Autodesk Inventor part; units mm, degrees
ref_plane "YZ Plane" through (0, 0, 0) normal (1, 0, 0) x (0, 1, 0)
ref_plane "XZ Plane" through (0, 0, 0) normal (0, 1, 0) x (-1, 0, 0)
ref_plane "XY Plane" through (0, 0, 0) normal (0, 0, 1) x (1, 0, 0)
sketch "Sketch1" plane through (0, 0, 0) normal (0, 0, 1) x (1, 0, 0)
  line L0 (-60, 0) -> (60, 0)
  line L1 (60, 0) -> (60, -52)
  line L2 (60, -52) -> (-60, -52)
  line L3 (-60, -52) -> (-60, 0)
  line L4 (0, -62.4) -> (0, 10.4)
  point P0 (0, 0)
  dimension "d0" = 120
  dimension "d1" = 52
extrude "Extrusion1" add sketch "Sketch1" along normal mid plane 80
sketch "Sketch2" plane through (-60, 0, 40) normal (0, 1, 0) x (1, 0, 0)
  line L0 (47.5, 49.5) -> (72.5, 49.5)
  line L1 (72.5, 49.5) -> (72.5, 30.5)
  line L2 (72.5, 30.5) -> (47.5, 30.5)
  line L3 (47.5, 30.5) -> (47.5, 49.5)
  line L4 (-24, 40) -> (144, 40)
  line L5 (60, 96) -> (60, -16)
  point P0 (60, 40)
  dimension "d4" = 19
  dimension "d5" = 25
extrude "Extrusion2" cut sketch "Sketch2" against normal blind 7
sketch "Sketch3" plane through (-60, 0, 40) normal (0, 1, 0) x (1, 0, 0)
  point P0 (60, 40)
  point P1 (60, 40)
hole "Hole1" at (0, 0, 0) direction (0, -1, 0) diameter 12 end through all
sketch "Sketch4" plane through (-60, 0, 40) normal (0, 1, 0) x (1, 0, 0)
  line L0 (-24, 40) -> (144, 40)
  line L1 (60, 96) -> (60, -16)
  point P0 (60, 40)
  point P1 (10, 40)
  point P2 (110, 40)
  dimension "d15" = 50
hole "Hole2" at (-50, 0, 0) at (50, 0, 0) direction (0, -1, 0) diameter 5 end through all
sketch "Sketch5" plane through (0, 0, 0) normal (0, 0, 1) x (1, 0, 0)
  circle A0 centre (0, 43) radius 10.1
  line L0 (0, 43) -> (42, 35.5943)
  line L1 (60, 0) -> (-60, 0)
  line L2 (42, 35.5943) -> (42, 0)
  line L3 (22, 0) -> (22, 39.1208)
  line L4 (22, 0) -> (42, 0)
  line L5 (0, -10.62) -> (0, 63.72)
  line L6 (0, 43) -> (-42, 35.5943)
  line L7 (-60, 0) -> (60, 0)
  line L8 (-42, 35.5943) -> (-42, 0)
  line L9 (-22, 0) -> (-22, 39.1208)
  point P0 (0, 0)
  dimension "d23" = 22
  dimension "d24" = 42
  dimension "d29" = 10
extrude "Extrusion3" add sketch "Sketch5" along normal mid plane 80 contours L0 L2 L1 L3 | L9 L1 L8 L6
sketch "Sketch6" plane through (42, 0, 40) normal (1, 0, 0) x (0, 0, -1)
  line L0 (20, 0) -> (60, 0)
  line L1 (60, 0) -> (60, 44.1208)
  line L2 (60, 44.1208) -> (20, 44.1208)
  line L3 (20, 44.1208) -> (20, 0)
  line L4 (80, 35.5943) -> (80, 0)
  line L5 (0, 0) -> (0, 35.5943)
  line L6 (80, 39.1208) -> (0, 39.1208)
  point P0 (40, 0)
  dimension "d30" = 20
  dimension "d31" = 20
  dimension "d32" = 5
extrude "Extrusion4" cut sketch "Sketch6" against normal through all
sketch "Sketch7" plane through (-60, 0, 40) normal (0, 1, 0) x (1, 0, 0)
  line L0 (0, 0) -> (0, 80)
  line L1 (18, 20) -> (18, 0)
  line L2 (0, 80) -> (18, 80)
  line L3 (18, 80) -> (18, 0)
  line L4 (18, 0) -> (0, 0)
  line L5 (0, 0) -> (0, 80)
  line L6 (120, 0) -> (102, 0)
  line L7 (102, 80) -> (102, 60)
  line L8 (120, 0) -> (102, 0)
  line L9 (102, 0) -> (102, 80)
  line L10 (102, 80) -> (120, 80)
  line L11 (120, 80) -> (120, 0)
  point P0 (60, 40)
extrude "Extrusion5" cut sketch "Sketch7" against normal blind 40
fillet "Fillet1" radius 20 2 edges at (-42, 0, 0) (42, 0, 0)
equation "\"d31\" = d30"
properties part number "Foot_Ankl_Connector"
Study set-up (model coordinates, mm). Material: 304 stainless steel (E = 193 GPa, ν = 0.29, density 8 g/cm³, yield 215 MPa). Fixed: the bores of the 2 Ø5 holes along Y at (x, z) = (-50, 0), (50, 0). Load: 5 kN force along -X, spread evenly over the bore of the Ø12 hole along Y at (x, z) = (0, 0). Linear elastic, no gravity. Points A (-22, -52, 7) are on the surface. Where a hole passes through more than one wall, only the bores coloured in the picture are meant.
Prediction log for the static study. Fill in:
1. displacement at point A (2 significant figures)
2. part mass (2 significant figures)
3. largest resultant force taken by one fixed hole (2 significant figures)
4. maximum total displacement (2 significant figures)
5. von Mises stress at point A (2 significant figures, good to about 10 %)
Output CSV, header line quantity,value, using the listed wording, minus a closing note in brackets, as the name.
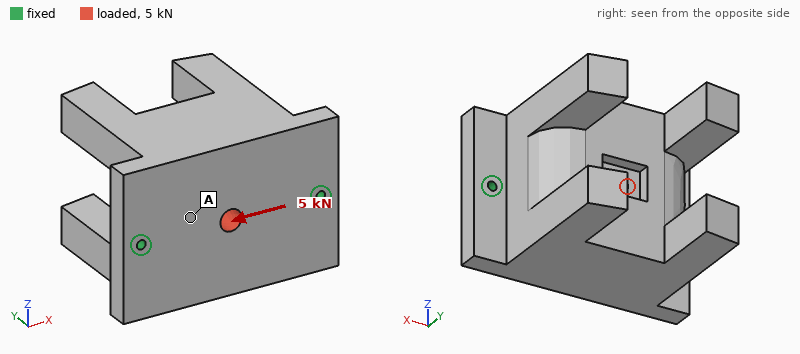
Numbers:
quantity,value
displacement at point A,0.89 µm
part mass,3.4 kg
largest resultant force taken by one fixed hole,2.6 kN
maximum total displacement,2.3 µm
von Mises stress at point A,2.7 MPa
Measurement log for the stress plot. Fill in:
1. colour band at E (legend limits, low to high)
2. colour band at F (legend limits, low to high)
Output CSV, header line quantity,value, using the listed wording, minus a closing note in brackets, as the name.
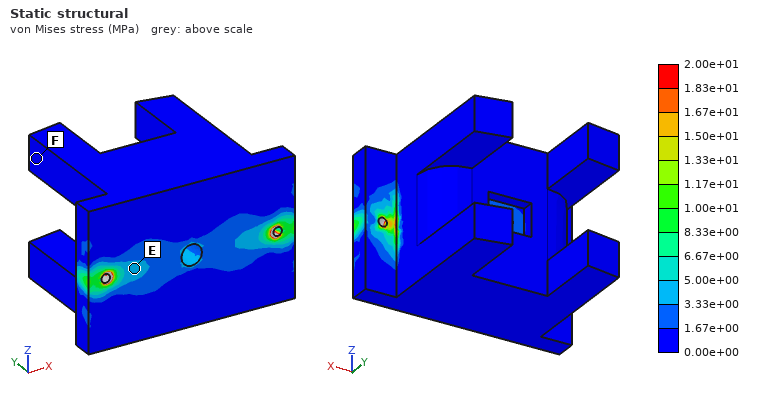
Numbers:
quantity,value
colour band at E,3.33e+00 to 5.00e+00 MPa
colour band at F,0.00e+00 to 1.67e+00 MPa
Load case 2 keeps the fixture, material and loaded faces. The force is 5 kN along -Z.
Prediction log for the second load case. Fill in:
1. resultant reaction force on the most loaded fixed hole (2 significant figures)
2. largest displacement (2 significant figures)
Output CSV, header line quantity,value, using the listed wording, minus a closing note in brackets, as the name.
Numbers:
quantity,value
resultant reaction force on the most loaded fixed hole,2.5 kN
largest displacement,43 µm
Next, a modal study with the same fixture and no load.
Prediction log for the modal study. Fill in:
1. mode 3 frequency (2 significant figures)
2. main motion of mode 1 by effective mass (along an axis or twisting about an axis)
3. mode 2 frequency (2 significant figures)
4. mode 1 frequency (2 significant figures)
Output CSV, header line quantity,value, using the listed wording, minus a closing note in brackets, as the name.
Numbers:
quantity,value
mode 3 frequency,3700 Hz
main motion of mode 1 by effective mass,along Z
mode 2 frequency,3700 Hz
mode 1 frequency,900 Hz
